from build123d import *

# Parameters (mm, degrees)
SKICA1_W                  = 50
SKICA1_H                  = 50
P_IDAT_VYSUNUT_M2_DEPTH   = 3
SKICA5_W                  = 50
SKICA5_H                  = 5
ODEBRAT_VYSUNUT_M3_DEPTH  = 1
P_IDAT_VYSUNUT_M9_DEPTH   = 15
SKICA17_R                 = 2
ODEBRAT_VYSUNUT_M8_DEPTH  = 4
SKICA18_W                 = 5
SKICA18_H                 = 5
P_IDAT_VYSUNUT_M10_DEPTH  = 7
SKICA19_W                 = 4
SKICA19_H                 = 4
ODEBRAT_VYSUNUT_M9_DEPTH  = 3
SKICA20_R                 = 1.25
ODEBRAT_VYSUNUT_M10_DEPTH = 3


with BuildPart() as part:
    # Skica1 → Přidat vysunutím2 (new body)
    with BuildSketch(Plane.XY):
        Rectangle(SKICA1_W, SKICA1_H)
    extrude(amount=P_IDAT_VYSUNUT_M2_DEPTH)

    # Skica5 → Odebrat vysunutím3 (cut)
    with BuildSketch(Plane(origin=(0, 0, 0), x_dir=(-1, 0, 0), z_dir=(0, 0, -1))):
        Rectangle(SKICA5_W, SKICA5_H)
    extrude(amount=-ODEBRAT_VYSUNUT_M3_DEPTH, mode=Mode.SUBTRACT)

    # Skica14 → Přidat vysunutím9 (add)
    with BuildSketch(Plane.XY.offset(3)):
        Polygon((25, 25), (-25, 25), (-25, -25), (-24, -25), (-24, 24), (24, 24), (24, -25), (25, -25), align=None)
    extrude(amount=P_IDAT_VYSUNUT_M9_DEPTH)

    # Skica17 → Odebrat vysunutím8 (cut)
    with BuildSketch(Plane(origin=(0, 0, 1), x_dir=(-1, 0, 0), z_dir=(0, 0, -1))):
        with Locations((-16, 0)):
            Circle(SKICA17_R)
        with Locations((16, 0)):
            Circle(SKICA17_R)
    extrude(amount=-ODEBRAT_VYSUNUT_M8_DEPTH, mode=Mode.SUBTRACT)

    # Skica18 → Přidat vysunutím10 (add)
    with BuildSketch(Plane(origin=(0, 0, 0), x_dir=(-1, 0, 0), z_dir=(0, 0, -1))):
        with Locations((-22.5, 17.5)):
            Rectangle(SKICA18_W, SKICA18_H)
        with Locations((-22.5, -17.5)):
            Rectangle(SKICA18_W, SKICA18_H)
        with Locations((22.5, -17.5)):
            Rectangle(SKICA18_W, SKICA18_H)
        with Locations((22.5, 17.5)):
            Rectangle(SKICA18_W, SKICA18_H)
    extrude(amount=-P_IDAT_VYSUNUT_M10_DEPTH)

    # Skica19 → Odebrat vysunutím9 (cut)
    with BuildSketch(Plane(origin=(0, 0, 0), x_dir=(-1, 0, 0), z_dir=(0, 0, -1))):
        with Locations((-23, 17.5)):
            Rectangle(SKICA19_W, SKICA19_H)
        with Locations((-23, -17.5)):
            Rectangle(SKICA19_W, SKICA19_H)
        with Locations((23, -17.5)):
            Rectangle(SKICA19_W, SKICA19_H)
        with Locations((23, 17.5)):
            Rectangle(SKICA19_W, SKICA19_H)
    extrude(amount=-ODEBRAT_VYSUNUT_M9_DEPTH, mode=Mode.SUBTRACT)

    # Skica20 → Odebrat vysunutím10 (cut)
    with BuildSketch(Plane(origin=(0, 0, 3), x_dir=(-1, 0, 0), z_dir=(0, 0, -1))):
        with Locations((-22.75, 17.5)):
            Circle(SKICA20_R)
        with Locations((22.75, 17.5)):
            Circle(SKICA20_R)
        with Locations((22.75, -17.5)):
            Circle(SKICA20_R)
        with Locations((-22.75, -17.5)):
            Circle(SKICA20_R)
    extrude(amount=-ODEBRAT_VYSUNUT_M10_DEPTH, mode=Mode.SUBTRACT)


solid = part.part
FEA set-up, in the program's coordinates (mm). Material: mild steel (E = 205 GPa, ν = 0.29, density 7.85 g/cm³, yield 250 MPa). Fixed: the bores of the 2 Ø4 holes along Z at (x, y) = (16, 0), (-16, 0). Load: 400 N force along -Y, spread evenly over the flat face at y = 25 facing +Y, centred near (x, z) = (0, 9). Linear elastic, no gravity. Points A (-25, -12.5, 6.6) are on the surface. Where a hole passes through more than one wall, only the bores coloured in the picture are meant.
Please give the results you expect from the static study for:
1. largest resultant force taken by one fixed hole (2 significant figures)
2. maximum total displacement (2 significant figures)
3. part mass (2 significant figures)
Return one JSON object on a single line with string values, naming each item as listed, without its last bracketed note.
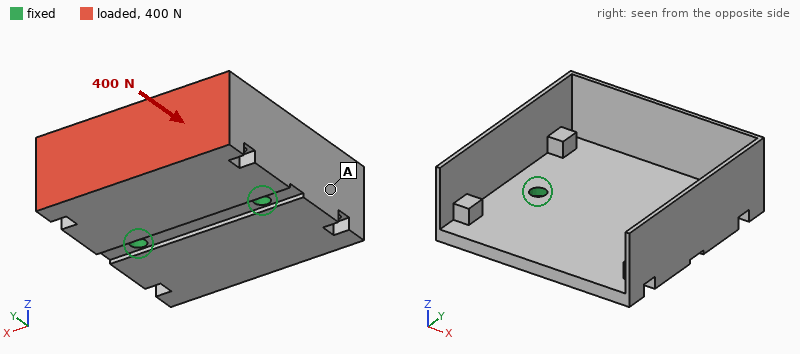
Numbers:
{"largest resultant force taken by one fixed hole": "200 N", "maximum total displacement": "0.13 mm", "part mass": "74 g"}
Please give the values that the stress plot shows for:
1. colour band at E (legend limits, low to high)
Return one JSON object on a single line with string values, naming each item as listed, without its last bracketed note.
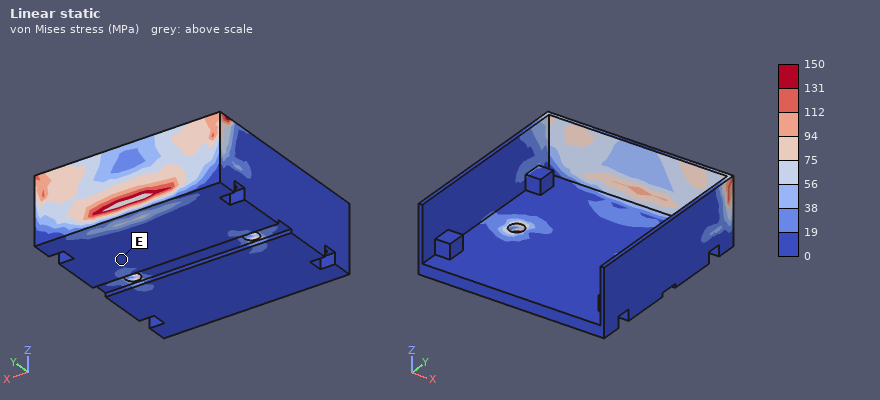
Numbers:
{"colour band at E": "0 to 19 MPa"}
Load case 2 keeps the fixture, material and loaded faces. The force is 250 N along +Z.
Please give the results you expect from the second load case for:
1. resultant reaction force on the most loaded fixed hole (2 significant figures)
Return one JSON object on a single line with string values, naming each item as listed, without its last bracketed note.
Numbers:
{"resultant reaction force on the most loaded fixed hole": "130 N"}
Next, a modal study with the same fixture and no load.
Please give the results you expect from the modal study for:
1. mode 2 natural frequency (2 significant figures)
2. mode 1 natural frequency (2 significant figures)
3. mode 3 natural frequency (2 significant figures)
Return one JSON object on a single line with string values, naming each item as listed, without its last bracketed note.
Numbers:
{"mode 2 natural frequency": "3300 Hz", "mode 1 natural frequency": "2200 Hz", "mode 3 natural frequency": "4200 Hz"}
